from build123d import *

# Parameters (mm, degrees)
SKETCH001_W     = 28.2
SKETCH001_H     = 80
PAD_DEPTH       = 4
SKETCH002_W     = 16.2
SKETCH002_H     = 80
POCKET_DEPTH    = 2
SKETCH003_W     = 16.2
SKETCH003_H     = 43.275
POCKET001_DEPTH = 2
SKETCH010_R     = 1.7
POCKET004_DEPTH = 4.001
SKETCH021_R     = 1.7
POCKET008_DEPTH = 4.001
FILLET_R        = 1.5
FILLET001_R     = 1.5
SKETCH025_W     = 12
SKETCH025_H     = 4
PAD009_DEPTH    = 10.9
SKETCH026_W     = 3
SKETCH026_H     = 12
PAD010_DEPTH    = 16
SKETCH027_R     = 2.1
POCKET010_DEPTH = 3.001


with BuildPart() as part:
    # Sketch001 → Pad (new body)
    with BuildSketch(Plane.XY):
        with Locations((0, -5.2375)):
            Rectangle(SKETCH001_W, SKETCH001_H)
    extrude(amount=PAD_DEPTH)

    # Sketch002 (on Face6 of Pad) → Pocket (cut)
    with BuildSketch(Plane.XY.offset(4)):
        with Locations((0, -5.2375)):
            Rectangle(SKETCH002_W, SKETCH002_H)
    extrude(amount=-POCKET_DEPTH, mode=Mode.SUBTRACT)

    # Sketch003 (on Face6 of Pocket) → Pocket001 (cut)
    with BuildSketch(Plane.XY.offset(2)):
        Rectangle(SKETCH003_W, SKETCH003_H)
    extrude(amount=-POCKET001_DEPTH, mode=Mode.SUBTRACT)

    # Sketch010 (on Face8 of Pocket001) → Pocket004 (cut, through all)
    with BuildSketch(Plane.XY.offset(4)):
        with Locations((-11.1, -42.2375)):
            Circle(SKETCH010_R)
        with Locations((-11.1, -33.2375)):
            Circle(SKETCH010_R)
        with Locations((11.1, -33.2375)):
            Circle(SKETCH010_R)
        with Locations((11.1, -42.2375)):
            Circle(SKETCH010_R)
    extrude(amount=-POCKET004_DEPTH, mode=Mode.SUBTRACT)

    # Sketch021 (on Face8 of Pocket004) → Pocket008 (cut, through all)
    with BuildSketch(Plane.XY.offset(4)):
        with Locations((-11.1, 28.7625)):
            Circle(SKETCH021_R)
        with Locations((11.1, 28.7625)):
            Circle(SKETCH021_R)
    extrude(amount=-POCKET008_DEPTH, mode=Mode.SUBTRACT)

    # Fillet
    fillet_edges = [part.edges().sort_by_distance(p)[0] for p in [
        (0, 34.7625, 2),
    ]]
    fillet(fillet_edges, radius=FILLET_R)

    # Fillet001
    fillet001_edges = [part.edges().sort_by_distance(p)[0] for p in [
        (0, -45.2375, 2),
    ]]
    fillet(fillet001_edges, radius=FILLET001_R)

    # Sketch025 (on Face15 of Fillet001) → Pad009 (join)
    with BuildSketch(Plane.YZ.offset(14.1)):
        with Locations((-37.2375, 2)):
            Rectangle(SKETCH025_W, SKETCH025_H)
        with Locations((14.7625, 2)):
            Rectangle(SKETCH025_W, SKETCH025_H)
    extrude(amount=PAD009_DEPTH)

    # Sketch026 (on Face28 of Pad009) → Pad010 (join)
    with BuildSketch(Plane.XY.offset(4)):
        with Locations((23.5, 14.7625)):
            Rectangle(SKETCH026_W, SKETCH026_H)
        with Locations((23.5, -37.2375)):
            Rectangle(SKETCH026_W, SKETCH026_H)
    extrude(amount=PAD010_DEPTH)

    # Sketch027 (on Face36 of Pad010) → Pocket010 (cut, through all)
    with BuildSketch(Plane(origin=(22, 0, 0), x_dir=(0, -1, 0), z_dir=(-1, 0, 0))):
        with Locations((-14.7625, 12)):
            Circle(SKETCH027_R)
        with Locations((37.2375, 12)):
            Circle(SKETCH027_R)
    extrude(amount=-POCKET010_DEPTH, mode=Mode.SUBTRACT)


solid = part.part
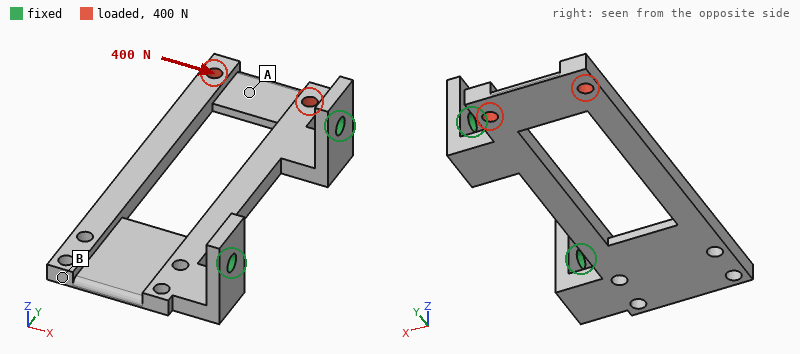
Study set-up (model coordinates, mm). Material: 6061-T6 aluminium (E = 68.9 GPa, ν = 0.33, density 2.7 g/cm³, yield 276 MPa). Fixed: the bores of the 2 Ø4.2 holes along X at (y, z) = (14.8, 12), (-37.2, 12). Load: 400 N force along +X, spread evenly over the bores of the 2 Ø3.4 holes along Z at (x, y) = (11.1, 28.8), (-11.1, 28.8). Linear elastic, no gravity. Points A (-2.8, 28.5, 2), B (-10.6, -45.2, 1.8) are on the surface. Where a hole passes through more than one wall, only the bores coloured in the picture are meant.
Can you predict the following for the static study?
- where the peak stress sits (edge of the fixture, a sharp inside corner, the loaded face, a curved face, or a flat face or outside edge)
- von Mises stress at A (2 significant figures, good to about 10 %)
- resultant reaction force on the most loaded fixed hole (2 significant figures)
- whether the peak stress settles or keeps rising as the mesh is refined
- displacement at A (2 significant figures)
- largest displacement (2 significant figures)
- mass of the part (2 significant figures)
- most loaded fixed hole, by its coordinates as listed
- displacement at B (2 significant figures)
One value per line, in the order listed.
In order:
edge of the fixture
29 MPa
480 N
keeps rising
0.23 mm
0.26 mm
19 g
(14.8, 12)
0.078 mm
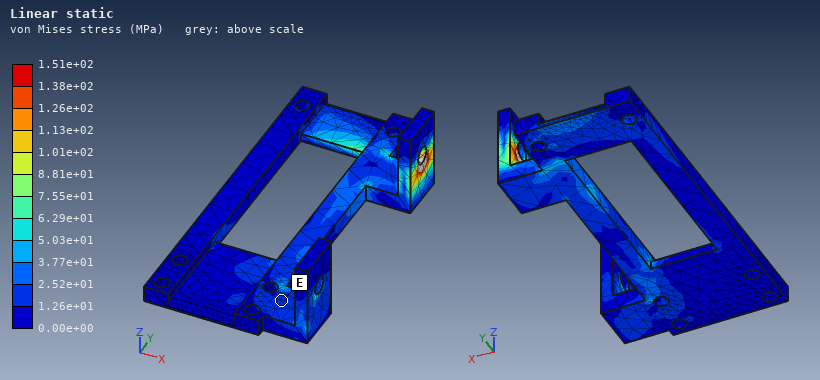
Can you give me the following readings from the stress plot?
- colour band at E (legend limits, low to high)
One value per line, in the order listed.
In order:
1.26e+01 to 2.52e+01 MPa
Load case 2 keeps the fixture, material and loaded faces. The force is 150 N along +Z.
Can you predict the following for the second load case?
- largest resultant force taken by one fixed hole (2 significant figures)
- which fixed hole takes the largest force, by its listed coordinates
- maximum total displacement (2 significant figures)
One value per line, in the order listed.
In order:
150 N
(14.8, 12)
1.0 mm
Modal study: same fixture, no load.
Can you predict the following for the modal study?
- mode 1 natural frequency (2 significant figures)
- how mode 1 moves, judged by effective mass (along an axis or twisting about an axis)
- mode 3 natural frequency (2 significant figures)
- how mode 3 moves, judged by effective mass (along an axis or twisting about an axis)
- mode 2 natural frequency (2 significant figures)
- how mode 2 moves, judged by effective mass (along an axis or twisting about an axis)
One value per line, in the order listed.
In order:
830 Hz
along Z
2900 Hz
along Y
1700 Hz
twisting about X
